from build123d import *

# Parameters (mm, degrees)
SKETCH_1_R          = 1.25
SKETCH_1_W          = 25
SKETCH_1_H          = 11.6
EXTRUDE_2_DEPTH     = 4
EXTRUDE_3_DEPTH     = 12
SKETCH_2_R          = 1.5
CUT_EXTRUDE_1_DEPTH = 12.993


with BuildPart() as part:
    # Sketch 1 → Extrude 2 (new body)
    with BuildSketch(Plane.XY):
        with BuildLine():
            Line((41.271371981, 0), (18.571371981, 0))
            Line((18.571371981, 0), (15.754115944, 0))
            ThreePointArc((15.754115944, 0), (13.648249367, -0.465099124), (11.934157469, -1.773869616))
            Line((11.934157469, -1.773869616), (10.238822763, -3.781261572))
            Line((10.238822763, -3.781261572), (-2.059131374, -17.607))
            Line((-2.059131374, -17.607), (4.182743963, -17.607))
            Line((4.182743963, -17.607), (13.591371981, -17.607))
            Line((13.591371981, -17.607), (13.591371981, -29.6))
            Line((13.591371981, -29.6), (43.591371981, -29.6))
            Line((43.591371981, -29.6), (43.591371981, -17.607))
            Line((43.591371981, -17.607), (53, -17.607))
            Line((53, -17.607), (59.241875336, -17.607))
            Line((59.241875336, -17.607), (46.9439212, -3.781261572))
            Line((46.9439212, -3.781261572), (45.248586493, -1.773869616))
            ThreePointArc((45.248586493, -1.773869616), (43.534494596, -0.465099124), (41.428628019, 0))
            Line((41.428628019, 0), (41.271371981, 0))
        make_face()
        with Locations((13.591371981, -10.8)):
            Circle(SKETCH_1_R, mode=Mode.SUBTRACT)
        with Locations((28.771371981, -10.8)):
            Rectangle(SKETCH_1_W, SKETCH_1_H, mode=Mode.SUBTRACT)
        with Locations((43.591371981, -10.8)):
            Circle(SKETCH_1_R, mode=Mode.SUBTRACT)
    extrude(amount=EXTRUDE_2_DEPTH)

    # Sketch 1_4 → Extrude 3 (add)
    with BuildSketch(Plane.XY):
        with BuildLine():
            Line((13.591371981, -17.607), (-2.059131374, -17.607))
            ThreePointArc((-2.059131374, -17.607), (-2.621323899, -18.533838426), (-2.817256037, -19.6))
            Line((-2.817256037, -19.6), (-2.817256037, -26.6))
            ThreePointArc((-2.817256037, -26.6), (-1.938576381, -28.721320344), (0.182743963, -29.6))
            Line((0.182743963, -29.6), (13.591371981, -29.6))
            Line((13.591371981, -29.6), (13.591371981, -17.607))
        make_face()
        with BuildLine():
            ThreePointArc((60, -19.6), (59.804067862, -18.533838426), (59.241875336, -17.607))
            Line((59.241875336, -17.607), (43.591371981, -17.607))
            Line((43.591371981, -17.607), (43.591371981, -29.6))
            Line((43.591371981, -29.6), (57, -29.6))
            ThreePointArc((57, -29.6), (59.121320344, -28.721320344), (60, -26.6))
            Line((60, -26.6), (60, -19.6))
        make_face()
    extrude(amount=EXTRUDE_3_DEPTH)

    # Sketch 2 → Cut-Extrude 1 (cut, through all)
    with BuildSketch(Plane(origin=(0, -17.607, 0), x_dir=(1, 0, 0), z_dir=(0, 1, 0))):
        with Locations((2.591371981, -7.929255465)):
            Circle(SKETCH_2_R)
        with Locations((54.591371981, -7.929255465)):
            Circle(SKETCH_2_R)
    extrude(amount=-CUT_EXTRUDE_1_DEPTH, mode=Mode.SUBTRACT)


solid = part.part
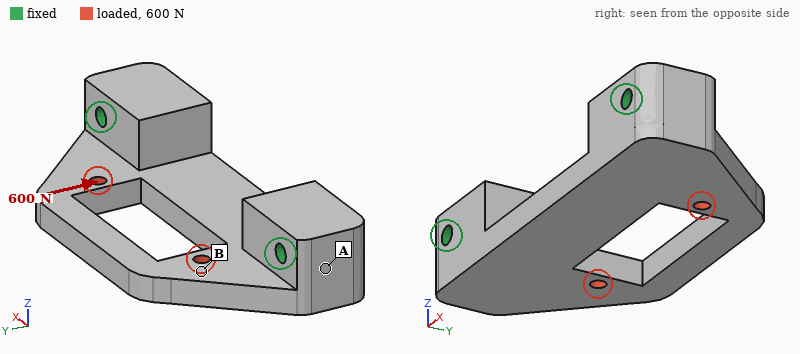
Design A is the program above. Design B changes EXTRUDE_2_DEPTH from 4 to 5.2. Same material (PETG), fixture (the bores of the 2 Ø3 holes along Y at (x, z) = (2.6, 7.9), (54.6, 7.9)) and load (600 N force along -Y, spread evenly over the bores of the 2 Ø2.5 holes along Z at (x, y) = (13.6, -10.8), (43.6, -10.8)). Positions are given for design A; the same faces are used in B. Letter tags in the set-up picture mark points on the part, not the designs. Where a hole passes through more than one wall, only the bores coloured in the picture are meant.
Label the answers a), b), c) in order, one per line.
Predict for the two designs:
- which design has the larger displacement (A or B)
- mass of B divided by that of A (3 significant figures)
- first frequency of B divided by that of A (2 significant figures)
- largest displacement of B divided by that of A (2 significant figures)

a) A
b) 1.13
c) 1.2
d) 0.80
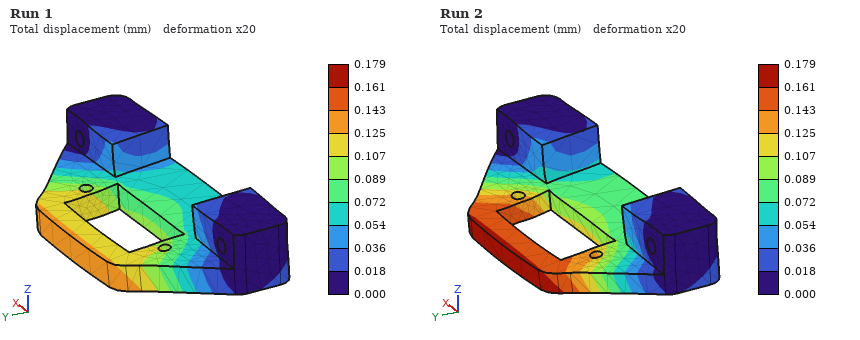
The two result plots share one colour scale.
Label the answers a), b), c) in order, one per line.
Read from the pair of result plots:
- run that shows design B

a) Run 1
